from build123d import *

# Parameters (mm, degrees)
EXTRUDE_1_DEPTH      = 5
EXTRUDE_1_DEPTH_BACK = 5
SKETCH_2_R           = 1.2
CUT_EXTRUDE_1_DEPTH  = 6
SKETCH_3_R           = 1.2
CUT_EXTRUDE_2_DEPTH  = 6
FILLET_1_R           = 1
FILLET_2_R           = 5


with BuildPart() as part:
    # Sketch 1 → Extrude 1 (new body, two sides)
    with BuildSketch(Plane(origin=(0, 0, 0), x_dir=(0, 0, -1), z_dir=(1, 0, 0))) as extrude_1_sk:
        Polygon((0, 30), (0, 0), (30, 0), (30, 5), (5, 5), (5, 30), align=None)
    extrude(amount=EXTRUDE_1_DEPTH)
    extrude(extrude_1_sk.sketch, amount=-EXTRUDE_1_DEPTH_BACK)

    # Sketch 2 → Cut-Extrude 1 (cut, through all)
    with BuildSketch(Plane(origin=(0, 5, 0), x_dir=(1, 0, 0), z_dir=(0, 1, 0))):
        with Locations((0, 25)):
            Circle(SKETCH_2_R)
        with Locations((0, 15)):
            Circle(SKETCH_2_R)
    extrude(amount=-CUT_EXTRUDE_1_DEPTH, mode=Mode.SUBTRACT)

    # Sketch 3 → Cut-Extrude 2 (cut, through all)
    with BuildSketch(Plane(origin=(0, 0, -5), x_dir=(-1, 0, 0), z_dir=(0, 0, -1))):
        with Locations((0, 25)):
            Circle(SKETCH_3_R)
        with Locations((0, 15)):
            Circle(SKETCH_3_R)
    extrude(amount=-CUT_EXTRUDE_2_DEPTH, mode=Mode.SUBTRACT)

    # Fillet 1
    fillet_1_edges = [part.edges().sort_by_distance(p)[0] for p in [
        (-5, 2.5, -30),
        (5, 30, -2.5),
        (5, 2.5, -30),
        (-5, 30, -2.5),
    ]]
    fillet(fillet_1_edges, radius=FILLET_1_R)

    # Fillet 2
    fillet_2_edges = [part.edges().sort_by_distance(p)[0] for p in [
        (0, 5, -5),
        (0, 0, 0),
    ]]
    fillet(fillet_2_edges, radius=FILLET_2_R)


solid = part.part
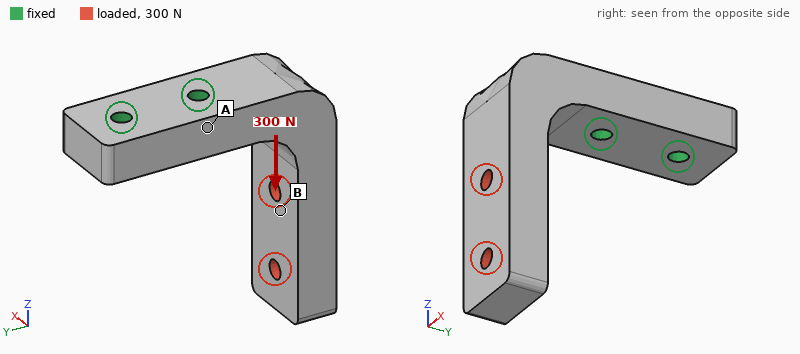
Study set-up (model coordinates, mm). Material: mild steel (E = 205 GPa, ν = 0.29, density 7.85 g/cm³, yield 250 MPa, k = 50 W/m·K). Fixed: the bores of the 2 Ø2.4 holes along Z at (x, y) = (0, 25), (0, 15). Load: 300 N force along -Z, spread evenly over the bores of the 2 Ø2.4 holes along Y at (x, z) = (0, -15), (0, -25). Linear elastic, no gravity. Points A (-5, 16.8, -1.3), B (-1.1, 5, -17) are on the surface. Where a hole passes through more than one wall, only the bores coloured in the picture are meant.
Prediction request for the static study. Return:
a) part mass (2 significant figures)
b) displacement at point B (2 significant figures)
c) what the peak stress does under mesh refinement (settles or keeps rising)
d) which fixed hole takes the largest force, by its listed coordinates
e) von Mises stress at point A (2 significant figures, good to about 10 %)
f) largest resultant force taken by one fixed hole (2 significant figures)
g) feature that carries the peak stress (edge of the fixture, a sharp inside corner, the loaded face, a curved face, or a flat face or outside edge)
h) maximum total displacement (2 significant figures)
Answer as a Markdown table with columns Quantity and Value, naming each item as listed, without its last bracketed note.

| Quantity | Value |
|---|---|
| part mass | 21 g |
| displacement at point B | 17 µm |
| what the peak stress does under mesh refinement | keeps rising |
| which fixed hole takes the largest force, by its listed coordinates | (0, 15) |
| von Mises stress at point A | 19 MPa |
| largest resultant force taken by one fixed hole | 390 N |
| feature that carries the peak stress | edge of the fixture |
| maximum total displacement | 33 µm |
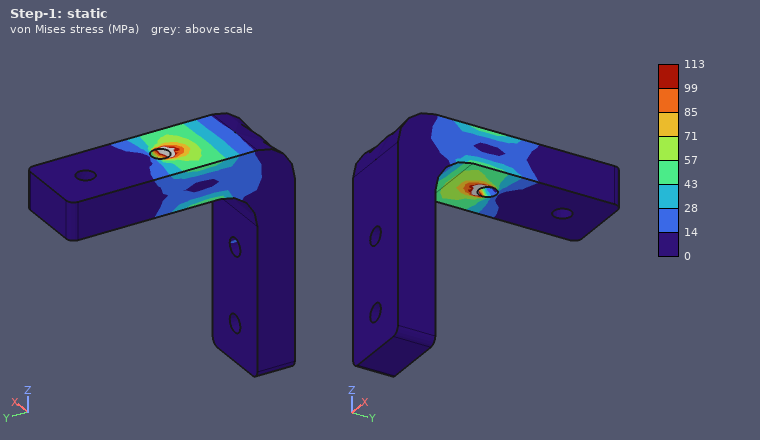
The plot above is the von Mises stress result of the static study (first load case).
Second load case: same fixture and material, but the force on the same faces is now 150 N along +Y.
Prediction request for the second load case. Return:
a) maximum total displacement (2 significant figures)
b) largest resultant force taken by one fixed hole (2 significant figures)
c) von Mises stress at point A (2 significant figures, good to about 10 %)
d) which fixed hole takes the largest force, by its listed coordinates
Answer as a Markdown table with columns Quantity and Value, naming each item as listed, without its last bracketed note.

| Quantity | Value |
|---|---|
| maximum total displacement | 50 µm |
| largest resultant force taken by one fixed hole | 150 N |
| von Mises stress at point A | 15 MPa |
| which fixed hole takes the largest force, by its listed coordinates | (0, 15) |
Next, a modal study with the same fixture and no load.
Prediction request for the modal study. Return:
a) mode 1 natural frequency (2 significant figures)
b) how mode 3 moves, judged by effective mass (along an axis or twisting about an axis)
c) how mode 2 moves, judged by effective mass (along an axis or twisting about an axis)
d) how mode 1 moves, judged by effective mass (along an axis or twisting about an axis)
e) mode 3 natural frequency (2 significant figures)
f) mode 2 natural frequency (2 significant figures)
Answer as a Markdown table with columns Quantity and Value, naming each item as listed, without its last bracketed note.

| Quantity | Value |
|---|---|
| mode 1 natural frequency | 3600 Hz |
| how mode 3 moves, judged by effective mass | along Z |
| how mode 2 moves, judged by effective mass | along X |
| how mode 1 moves, judged by effective mass | along Y |
| mode 3 natural frequency | 12 kHz |
| mode 2 natural frequency | 4400 Hz |
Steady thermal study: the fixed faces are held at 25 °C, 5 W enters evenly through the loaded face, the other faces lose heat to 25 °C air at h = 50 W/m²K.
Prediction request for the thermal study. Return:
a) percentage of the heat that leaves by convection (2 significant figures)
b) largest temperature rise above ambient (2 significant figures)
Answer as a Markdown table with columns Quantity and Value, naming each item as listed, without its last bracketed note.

| Quantity | Value |
|---|---|
| percentage of the heat that leaves by convection | 29 % |
| largest temperature rise above ambient | 41 K |
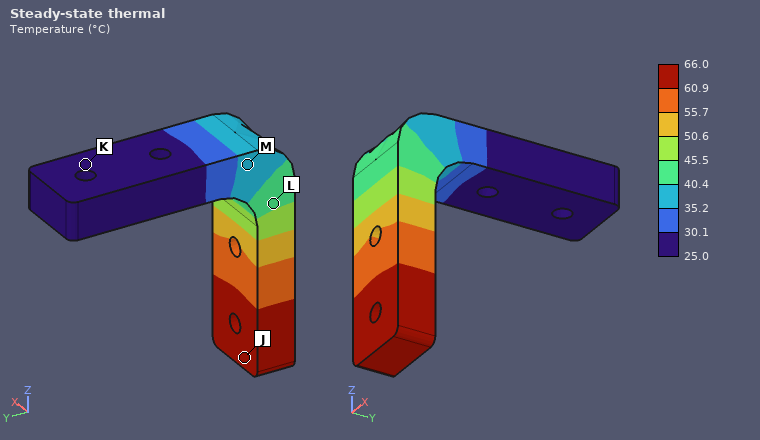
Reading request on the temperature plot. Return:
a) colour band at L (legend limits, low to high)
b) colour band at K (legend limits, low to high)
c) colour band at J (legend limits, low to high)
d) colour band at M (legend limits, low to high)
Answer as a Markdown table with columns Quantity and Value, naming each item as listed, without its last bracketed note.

| Quantity | Value |
|---|---|
| colour band at L | 40.4 to 45.5 °C |
| colour band at K | 25.0 to 30.1 °C |
| colour band at J | 60.9 to 66.0 °C |
| colour band at M | 35.2 to 40.4 °C |
